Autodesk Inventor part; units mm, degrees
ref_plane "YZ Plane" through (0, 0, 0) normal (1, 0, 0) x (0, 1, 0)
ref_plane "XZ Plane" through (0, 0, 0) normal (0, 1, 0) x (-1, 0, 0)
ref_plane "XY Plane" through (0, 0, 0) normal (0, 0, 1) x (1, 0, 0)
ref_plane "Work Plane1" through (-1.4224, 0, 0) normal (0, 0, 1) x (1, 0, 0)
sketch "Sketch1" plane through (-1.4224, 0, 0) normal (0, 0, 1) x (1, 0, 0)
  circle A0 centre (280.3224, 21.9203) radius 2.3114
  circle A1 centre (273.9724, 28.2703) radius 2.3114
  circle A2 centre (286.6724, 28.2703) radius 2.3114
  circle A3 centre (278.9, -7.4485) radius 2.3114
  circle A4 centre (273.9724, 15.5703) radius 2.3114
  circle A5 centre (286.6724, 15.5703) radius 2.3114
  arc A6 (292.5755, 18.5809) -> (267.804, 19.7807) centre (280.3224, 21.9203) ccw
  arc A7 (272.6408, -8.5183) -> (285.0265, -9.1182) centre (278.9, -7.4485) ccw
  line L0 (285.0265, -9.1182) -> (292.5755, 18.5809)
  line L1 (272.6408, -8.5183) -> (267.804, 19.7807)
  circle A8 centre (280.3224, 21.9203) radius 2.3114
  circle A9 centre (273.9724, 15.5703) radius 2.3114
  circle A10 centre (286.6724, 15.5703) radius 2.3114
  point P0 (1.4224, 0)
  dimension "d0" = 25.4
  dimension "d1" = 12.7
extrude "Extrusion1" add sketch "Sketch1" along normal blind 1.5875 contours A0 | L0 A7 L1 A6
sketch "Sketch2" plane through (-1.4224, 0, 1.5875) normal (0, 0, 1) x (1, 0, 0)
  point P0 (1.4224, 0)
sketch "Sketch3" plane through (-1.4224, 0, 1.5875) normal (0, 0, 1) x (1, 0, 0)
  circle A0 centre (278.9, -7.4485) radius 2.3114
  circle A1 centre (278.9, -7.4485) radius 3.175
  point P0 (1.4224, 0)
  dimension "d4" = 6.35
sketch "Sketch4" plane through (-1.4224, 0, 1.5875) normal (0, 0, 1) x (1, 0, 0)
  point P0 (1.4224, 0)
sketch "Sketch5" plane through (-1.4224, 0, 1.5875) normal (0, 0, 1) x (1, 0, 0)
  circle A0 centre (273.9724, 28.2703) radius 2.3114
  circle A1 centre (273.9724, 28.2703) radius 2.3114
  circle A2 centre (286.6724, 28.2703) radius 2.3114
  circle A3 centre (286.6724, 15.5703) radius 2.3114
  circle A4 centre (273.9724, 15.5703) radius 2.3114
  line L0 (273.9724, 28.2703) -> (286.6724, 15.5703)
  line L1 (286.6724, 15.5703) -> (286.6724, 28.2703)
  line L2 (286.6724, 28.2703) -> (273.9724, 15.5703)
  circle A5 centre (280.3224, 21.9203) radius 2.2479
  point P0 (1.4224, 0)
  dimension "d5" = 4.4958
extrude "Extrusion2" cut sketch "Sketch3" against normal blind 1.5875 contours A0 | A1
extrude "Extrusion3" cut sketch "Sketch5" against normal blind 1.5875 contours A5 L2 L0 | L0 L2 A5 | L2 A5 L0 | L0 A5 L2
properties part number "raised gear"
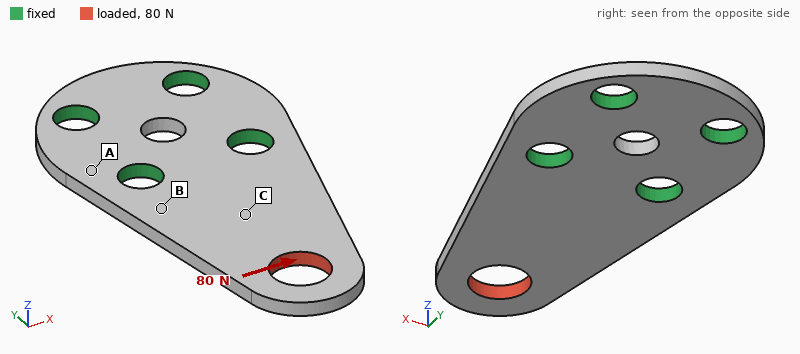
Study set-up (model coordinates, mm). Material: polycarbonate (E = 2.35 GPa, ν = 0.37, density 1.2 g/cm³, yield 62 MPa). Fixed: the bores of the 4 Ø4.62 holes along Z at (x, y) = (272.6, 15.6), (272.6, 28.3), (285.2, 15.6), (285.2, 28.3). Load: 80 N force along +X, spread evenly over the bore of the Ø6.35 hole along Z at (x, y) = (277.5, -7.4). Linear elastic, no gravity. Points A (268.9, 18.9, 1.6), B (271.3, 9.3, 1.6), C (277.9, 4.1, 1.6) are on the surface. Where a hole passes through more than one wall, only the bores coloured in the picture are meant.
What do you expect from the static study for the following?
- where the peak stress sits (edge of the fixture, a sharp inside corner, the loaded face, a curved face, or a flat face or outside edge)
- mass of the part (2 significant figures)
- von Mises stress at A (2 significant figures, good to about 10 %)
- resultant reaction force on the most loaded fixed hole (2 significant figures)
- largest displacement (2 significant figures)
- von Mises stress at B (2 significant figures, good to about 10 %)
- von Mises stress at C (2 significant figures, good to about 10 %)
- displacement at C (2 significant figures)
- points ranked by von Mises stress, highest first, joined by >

the loaded face
1.5 g
2.3 MPa
120 N
0.30 mm
9.3 MPa
6.0 MPa
0.056 mm
B > C > A
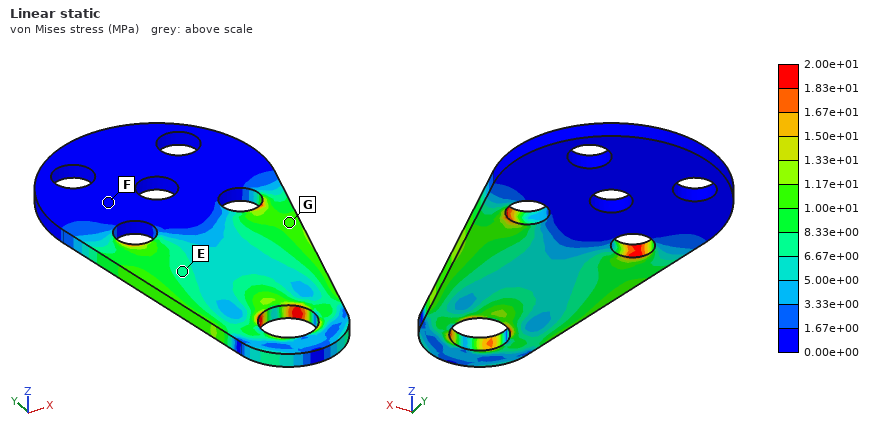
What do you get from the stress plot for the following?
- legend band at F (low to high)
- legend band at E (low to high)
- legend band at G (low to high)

0.00e+00 to 1.67e+00 MPa
6.67e+00 to 8.33e+00 MPa
1.00e+01 to 1.17e+01 MPa
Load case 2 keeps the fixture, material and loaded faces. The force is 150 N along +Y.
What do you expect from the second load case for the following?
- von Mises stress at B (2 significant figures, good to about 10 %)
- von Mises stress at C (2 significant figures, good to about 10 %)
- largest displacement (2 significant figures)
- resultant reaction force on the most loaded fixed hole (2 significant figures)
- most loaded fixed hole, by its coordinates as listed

6.0 MPa
5.0 MPa
93 µm
85 N
(272.6, 15.6)
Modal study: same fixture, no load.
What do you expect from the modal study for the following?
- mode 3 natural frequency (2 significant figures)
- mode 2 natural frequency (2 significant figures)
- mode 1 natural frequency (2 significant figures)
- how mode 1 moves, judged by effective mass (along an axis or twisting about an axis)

3100 Hz
2500 Hz
700 Hz
along Z
